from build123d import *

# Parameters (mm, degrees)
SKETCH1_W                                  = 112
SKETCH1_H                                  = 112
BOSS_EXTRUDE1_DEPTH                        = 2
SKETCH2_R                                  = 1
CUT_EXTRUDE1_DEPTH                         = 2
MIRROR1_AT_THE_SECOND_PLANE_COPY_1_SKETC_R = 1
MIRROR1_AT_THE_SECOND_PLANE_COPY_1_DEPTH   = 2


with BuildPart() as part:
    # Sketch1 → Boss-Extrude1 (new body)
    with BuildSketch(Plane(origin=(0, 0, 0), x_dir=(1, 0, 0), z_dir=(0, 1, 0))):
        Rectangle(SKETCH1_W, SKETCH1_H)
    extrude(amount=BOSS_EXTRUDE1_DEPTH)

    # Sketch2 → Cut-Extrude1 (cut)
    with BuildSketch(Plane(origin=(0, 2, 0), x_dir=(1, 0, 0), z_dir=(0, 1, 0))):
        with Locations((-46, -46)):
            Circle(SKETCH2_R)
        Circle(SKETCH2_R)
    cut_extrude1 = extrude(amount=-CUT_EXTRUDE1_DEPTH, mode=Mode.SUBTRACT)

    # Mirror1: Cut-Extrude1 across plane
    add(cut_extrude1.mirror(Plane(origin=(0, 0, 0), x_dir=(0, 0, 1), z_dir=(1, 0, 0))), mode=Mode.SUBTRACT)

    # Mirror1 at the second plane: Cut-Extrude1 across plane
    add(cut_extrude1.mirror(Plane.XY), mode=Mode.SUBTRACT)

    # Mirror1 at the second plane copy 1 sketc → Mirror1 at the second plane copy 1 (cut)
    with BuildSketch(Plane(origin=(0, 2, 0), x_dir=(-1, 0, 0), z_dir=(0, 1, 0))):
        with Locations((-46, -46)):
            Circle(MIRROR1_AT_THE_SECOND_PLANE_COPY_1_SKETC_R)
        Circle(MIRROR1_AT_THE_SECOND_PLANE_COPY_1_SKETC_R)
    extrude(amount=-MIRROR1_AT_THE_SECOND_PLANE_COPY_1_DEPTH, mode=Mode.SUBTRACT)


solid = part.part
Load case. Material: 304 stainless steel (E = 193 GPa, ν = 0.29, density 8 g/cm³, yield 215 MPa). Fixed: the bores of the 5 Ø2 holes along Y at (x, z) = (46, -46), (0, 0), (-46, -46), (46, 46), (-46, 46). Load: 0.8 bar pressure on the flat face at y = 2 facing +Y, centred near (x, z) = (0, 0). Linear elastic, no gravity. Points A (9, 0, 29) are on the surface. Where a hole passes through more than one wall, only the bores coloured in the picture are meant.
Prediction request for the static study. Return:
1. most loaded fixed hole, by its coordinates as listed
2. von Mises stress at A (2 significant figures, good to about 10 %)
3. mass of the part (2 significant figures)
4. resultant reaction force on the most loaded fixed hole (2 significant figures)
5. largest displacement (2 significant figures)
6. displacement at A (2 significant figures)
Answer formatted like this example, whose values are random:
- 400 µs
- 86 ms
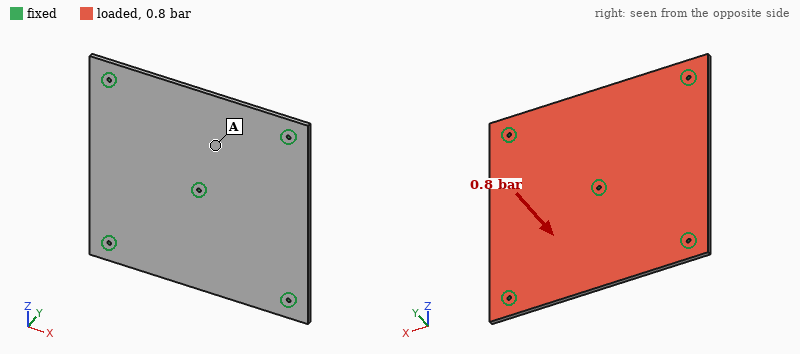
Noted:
- (0, 0)
- 21 MPa
- 200 g
- 370 N
- 93 µm
- 58 µm
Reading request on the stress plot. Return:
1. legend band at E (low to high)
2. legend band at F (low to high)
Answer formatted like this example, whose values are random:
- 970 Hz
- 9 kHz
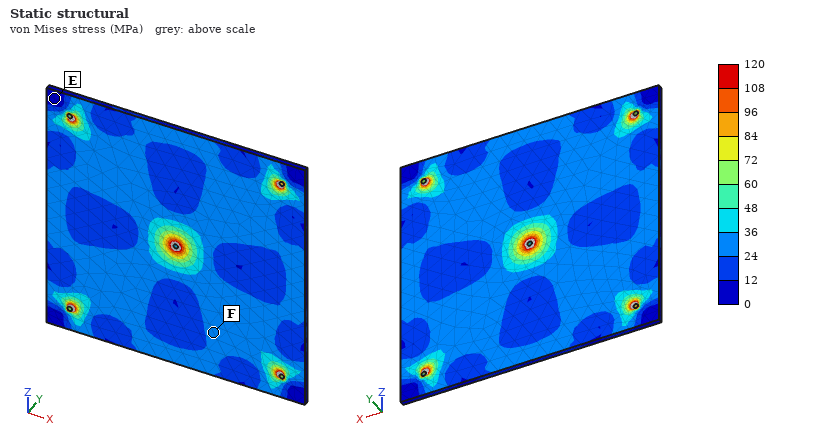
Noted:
- 0 to 12 MPa
- 24 to 36 MPa
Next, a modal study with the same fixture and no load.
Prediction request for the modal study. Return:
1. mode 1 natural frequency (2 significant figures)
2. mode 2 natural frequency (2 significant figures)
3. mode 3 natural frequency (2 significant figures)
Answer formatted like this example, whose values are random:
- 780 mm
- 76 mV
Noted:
- 1300 Hz
- 1300 Hz
- 1300 Hz
